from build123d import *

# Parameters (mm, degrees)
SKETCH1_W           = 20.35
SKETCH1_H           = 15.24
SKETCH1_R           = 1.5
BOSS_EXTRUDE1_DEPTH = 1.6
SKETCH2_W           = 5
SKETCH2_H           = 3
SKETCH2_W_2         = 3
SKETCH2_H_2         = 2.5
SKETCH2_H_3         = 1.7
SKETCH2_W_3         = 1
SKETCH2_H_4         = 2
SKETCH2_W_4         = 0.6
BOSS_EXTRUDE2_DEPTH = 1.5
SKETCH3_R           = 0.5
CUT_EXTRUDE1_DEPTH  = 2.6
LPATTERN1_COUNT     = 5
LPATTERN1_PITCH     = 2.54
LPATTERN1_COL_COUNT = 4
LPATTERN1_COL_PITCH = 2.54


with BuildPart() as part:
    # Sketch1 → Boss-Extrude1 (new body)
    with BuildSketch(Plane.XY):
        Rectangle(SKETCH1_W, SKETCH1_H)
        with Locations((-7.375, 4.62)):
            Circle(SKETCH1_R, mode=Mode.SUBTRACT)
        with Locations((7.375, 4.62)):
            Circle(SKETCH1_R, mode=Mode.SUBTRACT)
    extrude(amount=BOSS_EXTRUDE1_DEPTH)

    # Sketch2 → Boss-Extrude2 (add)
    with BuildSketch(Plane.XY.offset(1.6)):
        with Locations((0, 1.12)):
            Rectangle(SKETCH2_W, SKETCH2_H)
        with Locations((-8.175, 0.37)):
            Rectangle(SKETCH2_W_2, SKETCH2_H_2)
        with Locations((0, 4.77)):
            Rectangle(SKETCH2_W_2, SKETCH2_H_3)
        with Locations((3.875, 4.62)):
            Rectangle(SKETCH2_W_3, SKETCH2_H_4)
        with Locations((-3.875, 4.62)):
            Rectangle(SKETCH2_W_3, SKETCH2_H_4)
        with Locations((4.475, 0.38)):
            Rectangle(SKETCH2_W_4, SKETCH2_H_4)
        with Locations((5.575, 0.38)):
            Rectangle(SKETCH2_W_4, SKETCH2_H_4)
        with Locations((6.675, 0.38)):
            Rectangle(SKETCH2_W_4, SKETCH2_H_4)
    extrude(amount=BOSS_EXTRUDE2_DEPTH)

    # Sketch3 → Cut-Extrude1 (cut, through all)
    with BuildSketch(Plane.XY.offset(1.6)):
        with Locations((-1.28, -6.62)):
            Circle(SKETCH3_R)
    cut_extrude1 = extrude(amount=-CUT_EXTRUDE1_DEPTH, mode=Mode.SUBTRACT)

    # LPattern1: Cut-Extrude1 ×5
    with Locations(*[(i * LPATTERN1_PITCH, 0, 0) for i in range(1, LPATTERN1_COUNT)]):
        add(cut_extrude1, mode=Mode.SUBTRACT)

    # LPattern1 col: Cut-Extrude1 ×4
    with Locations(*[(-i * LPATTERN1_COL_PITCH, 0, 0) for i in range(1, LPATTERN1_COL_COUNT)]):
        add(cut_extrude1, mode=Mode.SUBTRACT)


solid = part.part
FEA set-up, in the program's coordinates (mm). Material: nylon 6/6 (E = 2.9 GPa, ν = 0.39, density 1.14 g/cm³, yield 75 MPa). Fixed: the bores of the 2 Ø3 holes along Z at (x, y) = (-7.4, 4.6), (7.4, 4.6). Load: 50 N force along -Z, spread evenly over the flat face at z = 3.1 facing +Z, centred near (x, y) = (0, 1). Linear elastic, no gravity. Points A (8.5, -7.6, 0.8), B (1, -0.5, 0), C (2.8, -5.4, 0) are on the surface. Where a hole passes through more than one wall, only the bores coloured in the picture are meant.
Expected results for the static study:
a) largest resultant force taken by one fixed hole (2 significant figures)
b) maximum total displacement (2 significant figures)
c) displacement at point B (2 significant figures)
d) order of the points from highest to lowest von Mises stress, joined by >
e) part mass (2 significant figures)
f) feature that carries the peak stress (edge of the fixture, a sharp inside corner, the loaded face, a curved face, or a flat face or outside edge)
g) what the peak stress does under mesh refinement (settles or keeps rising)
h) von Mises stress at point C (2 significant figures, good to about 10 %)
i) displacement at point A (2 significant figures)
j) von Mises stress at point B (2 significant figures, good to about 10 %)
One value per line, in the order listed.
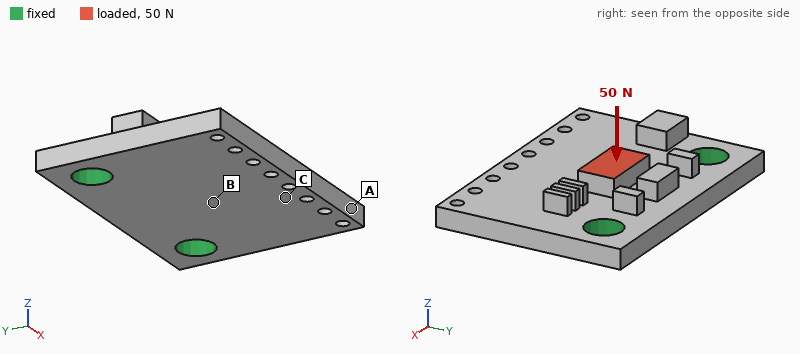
26 N
0.22 mm
0.11 mm
B > C > A
0.59 g
edge of the fixture
keeps rising
5.0 MPa
0.16 mm
8.6 MPa
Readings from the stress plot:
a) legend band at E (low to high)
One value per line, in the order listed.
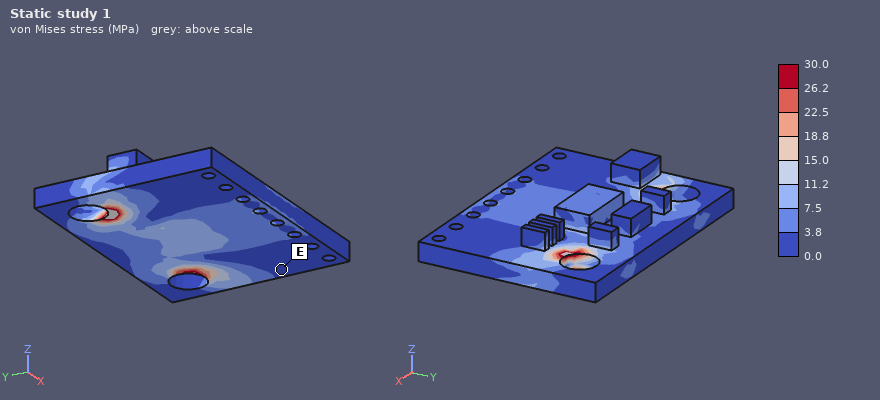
0.0 to 3.8 MPa
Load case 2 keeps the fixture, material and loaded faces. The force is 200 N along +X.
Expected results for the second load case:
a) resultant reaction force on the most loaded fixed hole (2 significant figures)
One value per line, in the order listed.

120 N
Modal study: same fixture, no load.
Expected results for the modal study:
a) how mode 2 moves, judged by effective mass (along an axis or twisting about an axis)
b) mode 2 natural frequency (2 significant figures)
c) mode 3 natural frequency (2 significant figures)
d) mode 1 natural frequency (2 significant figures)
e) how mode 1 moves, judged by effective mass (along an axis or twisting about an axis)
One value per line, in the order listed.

twisting about Y
5500 Hz
9700 Hz
3200 Hz
along Z
